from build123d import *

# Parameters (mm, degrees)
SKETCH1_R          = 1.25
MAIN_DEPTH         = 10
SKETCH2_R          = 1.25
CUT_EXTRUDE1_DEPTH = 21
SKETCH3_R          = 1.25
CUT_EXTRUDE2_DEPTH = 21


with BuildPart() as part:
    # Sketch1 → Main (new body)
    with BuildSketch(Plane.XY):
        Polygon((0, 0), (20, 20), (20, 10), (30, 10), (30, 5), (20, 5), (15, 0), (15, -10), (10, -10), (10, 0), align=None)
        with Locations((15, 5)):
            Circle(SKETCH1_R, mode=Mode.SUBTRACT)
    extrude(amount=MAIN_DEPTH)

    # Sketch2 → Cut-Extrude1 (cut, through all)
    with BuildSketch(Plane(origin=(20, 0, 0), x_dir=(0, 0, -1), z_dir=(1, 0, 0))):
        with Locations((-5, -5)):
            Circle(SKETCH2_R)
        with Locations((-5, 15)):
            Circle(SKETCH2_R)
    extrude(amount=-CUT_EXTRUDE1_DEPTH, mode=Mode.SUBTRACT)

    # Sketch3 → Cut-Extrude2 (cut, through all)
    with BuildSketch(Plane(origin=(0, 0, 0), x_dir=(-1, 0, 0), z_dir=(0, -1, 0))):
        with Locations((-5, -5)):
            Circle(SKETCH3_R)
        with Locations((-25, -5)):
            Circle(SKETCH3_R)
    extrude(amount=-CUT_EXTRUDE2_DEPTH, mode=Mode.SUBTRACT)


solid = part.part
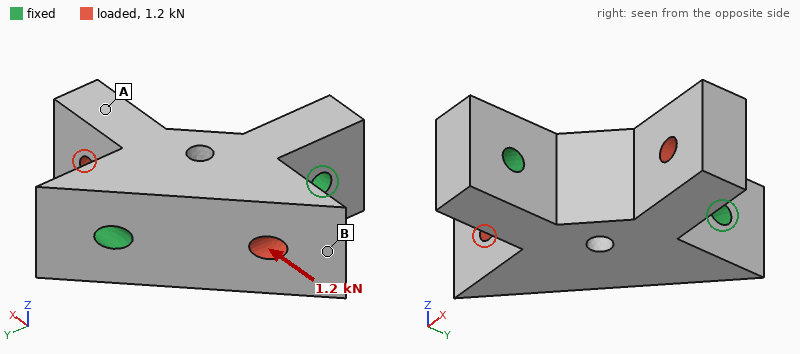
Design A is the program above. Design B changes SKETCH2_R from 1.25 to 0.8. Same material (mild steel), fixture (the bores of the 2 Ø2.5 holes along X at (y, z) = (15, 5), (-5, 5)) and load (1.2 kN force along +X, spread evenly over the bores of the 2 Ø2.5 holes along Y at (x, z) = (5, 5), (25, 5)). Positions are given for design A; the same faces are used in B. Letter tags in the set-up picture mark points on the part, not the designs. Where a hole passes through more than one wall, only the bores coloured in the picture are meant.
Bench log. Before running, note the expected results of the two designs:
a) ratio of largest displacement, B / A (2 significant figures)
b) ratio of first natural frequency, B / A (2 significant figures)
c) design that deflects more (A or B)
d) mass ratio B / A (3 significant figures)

1.1
0.88
B
1.01
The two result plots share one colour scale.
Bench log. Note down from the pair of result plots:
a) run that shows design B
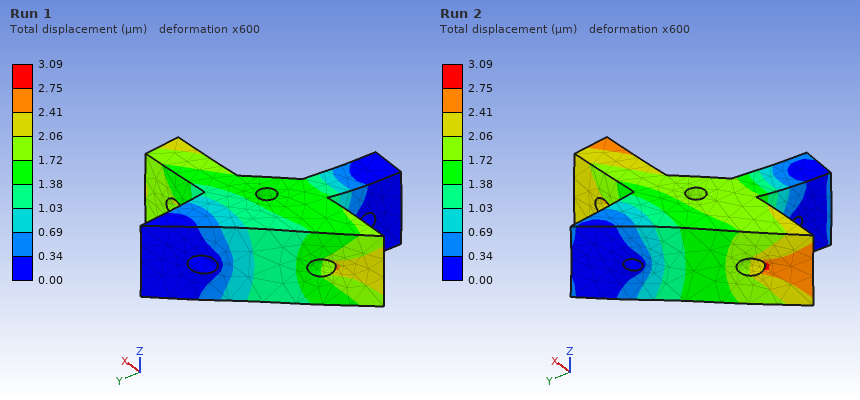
Run 2
